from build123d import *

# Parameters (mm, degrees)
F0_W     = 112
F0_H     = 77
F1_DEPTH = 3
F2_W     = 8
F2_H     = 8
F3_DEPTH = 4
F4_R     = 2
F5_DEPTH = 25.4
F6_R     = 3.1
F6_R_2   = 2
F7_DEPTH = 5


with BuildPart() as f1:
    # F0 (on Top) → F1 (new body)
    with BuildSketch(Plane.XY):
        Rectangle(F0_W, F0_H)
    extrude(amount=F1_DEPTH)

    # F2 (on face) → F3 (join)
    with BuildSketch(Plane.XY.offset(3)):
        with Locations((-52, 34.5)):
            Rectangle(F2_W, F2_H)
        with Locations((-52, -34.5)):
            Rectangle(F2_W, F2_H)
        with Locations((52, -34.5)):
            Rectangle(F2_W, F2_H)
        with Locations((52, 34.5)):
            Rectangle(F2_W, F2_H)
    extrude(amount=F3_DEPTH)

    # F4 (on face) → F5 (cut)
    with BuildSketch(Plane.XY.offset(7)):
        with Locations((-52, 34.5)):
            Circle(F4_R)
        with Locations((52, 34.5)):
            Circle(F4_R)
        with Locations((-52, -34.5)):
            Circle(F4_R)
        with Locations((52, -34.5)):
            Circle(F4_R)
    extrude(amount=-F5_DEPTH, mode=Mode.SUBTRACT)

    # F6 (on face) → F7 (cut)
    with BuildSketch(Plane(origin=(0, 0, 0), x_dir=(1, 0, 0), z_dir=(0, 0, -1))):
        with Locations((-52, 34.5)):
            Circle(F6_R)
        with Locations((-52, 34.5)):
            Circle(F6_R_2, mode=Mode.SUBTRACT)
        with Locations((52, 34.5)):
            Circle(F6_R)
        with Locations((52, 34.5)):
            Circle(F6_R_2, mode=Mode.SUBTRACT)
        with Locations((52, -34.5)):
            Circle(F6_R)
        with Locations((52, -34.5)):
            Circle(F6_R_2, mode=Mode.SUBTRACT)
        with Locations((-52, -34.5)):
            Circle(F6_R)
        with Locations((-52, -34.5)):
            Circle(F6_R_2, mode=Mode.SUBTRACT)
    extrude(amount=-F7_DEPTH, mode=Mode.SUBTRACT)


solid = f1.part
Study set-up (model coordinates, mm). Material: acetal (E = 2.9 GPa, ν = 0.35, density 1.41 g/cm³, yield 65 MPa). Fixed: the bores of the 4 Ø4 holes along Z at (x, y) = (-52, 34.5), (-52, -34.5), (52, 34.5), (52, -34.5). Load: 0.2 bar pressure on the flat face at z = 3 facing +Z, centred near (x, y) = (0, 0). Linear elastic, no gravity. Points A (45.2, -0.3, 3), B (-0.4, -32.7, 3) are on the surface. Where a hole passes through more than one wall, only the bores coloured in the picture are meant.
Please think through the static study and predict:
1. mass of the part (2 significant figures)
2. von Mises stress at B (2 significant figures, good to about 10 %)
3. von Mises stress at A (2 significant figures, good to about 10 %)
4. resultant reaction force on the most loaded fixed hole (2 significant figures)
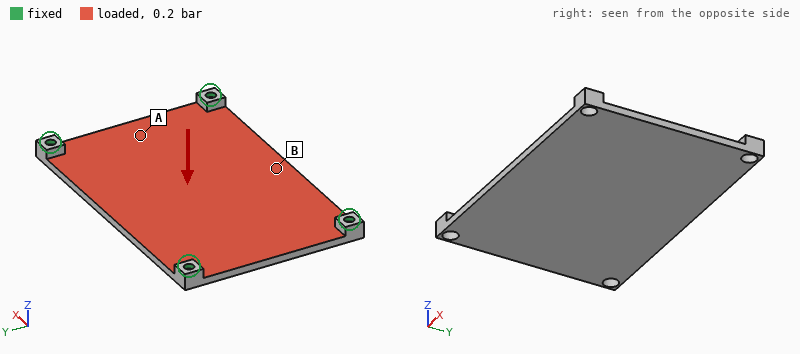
37 g
7.4 MPa
3.7 MPa
94 N
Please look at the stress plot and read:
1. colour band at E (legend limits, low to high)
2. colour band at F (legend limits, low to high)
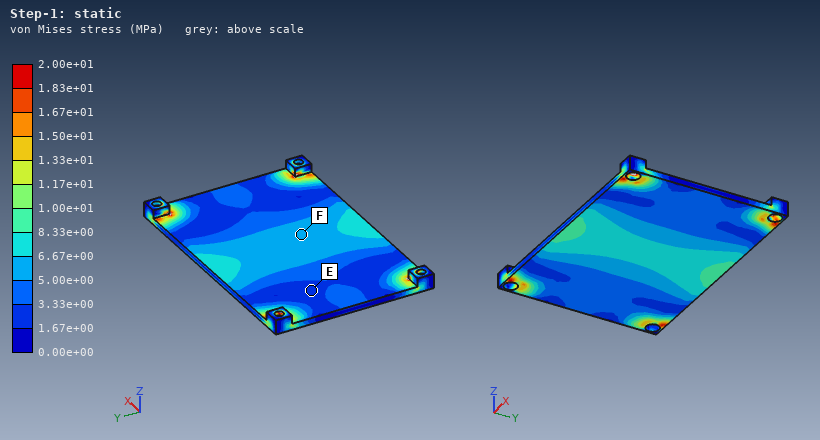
1.67e+00 to 3.33e+00 MPa
5.00e+00 to 6.67e+00 MPa
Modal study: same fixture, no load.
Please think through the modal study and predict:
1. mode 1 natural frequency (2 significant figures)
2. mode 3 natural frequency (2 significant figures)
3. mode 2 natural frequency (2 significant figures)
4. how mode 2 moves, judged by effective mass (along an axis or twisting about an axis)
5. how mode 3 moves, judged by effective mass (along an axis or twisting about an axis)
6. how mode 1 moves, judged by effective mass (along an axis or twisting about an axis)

320 Hz
780 Hz
530 Hz
twisting about X
twisting about Y
along Z
